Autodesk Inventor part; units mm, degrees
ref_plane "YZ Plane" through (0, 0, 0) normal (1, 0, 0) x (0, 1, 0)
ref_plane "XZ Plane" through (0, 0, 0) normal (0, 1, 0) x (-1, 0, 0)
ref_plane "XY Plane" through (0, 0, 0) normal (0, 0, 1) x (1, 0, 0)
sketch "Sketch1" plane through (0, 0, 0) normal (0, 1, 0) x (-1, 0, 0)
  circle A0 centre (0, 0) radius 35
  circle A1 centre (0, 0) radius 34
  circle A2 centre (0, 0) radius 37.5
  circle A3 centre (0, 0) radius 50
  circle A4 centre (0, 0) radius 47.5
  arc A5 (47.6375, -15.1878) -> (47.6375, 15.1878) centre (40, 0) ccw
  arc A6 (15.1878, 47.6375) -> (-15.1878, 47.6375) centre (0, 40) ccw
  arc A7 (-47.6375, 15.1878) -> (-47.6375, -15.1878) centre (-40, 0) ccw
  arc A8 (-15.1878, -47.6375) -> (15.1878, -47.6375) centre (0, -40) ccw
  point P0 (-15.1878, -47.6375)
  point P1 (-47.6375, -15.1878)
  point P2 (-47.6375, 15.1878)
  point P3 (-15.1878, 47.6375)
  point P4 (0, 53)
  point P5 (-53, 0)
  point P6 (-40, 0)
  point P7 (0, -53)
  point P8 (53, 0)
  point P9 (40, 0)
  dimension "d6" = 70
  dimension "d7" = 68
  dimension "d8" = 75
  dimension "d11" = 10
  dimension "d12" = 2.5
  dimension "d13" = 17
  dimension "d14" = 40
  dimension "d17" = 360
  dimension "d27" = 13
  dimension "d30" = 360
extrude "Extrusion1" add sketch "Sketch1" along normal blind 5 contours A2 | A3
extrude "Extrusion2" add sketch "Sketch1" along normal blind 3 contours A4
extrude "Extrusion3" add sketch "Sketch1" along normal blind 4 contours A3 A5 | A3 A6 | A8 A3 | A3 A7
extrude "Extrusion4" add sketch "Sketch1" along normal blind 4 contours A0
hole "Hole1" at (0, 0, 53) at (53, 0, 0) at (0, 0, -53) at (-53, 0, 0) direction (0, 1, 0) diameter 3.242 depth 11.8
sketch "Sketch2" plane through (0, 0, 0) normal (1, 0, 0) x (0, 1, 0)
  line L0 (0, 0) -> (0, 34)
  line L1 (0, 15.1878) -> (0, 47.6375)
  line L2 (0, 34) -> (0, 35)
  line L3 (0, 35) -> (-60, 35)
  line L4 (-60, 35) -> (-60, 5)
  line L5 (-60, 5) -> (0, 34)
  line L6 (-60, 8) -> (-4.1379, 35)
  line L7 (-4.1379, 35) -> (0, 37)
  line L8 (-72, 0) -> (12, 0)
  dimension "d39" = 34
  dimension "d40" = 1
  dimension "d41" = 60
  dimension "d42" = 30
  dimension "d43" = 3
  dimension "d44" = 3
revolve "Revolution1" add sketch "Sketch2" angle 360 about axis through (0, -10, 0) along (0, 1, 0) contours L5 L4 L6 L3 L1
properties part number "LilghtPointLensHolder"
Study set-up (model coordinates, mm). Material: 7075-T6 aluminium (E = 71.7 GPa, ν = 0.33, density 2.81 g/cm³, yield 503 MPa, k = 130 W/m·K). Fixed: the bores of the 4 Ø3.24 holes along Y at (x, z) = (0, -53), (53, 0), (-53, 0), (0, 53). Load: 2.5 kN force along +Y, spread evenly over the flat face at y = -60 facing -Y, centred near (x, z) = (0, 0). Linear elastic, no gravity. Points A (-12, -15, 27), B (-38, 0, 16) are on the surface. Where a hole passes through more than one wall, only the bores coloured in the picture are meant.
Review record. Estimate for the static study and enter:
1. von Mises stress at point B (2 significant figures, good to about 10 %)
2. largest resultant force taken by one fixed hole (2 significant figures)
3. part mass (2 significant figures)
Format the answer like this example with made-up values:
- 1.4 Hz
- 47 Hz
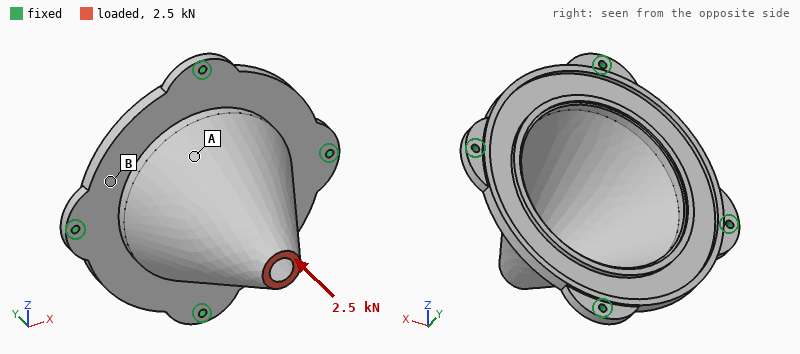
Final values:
- 30 MPa
- 790 N
- 110 g
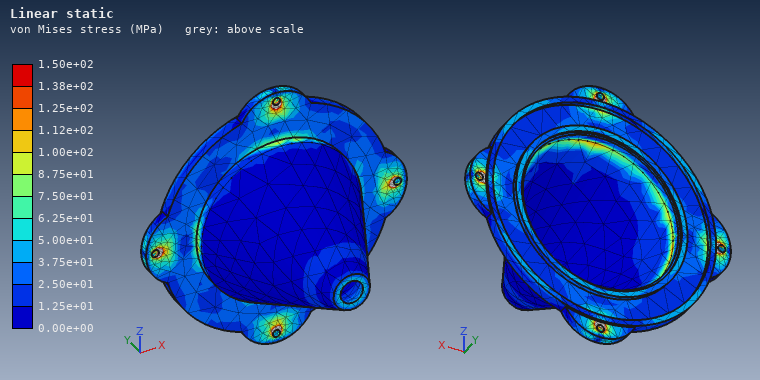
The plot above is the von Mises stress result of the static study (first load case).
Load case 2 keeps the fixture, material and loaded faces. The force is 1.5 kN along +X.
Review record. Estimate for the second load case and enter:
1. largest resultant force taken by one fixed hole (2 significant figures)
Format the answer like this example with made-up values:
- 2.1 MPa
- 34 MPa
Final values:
- 1.3 kN
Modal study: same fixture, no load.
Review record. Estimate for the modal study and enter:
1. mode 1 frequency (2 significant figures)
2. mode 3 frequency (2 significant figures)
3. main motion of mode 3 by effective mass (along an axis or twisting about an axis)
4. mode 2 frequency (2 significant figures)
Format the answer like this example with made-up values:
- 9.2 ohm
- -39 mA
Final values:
- 2400 Hz
- 2600 Hz
- along Y
- 2400 Hz
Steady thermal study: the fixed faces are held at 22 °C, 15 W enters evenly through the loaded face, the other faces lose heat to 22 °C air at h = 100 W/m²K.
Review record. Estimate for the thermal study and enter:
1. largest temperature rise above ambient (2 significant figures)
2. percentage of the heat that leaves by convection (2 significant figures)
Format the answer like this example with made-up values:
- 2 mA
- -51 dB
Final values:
- 22 K
- 76 %
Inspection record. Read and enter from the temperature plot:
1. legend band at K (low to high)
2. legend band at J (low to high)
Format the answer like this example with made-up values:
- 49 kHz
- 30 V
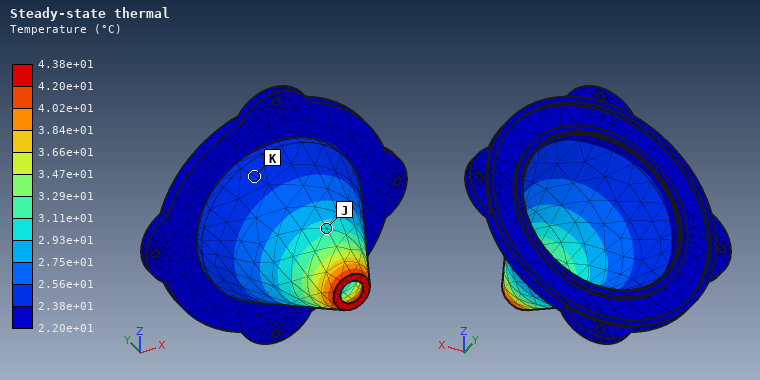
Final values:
- 2.38e+01 to 2.56e+01 °C
- 2.93e+01 to 3.11e+01 °C
